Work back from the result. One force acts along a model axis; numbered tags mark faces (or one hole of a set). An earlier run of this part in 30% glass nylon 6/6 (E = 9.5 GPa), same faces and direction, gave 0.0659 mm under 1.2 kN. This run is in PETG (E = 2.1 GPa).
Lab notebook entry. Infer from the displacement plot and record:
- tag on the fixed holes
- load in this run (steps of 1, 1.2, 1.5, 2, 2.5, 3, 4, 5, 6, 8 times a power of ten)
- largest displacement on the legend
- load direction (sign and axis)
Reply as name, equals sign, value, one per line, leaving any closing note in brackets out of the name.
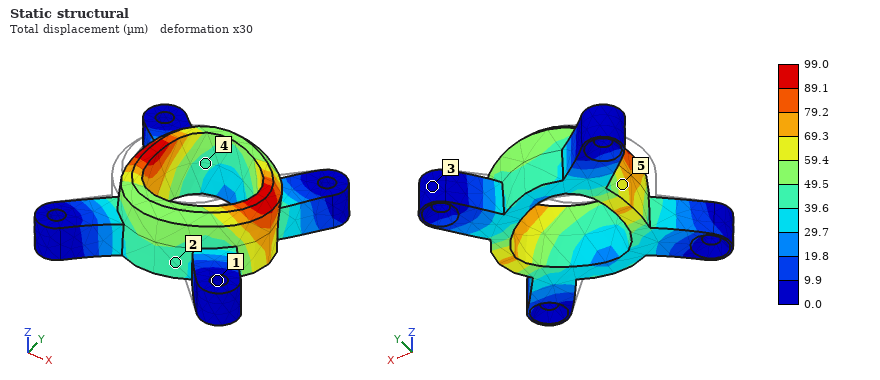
tag on the fixed holes = 1
load in this run = 400 N
largest displacement on the legend = 99.0 µm
load direction = +X
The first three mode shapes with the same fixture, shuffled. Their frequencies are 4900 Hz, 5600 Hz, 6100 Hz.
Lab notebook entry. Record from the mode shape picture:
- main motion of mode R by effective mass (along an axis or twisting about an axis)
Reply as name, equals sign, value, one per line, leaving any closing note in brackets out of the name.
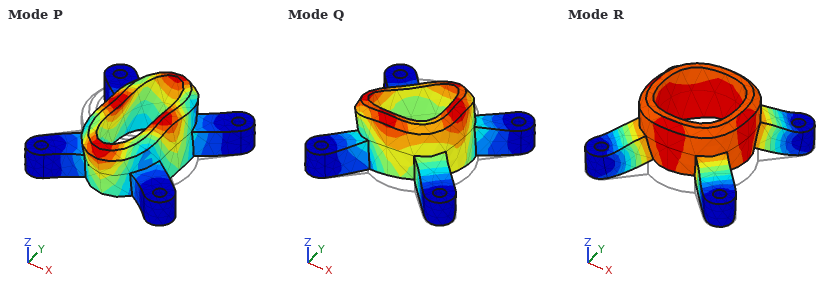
main motion of mode R by effective mass = along Z
